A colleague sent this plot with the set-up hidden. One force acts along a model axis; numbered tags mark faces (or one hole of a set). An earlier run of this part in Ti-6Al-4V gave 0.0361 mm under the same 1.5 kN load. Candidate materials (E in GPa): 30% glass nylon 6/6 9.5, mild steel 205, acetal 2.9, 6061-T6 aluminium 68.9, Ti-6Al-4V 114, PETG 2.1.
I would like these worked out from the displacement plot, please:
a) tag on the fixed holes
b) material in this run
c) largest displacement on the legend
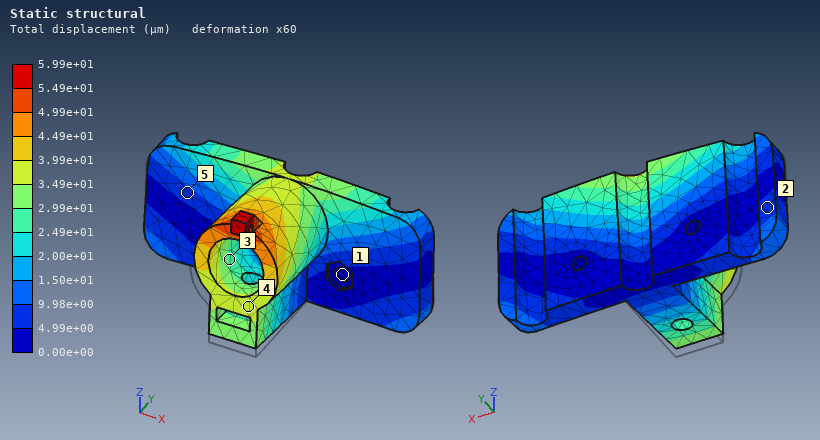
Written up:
1
6061-T6 aluminium
5.99e+01 µm
